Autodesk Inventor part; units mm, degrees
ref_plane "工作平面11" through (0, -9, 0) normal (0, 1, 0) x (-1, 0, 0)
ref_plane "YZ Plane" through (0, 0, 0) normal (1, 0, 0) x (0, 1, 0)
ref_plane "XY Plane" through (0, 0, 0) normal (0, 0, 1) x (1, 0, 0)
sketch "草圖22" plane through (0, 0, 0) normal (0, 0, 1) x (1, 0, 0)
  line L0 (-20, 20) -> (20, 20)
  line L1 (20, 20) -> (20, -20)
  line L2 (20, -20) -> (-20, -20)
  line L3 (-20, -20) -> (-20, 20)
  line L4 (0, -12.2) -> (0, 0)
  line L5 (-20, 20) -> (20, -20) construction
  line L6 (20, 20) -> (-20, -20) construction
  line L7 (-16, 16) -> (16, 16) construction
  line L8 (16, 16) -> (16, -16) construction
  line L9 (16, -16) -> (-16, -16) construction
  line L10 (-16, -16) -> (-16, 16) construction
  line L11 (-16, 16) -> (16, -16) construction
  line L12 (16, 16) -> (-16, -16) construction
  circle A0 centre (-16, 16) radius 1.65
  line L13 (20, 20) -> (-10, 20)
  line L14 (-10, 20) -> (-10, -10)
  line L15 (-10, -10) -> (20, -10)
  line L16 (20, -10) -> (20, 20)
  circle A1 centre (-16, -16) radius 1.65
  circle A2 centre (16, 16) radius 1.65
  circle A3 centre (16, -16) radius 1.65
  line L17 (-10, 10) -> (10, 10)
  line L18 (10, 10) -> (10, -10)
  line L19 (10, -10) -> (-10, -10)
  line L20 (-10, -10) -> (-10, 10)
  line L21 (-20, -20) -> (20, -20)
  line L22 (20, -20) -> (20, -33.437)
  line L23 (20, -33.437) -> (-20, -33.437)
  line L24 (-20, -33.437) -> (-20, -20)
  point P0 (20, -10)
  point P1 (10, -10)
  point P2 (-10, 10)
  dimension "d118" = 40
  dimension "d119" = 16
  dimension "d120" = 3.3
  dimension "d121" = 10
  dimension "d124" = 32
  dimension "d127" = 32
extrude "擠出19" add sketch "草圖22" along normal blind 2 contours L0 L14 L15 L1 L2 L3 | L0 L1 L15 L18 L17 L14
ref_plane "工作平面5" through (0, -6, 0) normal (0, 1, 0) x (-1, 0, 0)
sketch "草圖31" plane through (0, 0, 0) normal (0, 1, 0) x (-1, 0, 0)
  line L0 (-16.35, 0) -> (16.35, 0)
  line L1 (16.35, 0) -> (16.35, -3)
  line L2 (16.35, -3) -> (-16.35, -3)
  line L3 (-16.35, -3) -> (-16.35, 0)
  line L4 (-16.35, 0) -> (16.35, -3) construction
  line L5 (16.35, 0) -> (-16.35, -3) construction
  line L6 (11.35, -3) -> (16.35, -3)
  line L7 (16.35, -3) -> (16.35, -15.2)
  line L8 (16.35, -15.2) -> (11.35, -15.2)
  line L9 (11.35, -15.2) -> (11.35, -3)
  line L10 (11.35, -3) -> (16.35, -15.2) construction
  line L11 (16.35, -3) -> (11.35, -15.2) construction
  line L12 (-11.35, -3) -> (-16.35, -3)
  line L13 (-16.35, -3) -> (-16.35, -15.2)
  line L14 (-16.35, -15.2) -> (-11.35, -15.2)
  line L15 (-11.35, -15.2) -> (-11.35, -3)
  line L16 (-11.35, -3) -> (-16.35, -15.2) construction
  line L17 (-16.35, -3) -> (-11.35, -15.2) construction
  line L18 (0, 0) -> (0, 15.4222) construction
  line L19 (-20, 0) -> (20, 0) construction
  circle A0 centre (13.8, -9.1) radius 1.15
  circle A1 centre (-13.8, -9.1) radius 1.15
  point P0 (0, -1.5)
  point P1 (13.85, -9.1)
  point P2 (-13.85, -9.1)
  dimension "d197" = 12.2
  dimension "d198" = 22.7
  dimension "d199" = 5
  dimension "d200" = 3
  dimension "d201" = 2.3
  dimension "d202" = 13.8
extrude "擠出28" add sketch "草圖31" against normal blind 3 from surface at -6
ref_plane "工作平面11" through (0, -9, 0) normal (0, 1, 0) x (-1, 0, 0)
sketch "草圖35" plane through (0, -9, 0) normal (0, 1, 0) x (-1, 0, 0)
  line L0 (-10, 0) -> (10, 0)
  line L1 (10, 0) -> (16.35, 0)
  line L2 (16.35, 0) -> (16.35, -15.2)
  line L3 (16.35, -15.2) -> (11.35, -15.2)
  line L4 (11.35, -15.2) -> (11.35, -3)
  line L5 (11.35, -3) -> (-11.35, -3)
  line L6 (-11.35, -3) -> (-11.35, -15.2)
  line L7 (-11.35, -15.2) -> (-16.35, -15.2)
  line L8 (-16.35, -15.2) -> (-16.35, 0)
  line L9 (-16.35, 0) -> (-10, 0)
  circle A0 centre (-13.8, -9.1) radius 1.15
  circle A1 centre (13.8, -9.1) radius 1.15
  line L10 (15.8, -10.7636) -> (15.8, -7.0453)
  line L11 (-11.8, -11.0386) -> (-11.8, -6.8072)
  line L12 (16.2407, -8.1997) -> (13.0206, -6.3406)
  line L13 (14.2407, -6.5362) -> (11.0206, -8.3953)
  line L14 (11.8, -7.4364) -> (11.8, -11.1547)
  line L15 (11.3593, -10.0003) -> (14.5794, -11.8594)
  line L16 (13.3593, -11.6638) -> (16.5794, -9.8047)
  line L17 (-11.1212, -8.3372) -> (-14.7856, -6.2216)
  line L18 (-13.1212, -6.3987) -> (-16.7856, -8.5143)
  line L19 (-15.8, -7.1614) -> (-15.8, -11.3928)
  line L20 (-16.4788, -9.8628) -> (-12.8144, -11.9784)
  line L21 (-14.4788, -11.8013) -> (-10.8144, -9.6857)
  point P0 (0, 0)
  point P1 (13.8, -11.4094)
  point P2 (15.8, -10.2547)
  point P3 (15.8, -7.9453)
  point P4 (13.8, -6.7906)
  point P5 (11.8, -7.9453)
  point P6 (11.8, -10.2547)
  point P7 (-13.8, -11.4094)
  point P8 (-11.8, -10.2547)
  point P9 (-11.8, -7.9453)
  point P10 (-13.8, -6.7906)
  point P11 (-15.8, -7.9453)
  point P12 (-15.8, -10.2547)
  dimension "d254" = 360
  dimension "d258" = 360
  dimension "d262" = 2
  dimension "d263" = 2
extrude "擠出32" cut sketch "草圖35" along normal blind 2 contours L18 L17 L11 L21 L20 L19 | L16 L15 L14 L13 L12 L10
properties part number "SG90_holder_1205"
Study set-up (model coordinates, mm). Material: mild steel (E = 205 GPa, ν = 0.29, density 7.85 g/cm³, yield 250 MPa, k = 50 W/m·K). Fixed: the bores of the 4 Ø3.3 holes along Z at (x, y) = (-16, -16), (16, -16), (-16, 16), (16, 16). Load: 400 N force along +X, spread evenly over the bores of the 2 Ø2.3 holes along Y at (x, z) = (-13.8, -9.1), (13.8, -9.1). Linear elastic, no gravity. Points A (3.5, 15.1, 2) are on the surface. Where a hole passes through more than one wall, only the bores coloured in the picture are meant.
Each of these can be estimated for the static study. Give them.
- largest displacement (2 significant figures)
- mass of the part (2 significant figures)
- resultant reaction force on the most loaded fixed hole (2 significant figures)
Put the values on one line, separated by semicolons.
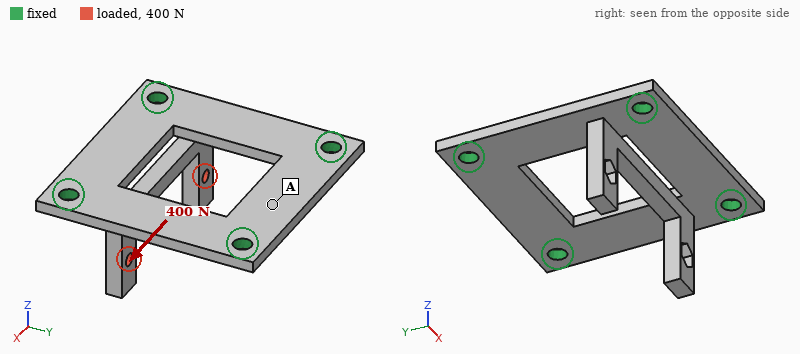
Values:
47 µm; 23 g; 190 N
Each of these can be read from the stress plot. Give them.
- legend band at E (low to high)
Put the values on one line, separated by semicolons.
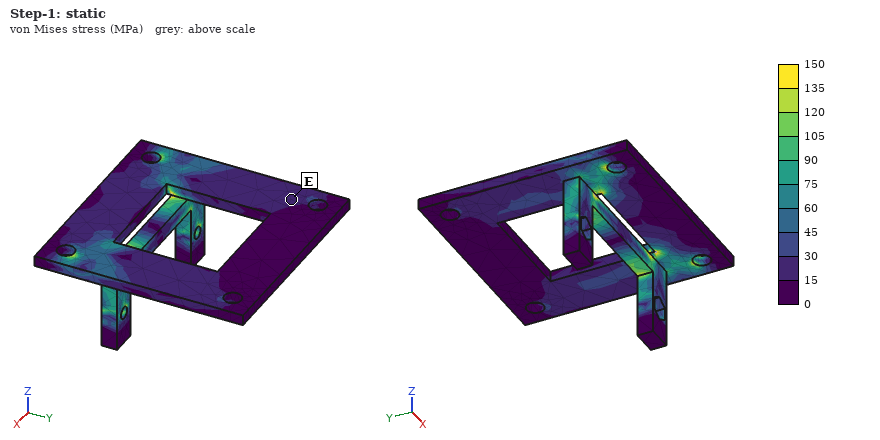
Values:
15 to 30 MPa
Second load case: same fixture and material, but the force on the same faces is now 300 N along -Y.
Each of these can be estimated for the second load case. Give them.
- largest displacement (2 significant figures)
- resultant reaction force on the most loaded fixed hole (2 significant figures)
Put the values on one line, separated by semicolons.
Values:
78 µm; 120 N
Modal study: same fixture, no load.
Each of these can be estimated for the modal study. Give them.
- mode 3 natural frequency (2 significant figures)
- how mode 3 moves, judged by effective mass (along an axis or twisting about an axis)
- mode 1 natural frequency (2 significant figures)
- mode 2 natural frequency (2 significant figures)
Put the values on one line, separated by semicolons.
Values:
9600 Hz; along Z; 6500 Hz; 7200 Hz
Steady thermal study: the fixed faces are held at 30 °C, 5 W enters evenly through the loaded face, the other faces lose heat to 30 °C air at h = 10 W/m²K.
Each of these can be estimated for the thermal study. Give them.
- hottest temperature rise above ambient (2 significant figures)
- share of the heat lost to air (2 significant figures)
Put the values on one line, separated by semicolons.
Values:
58 K; 7.6 %
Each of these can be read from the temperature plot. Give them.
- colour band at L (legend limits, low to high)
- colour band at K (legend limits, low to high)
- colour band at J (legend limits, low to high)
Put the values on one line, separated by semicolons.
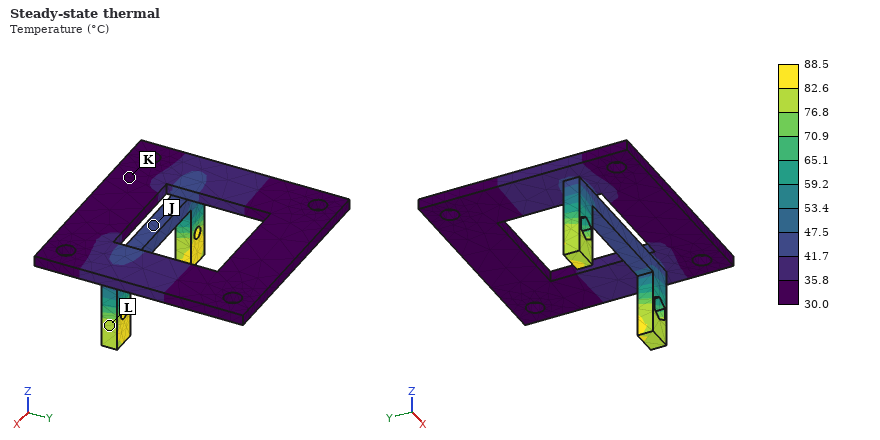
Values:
76.8 to 82.6 °C; 30.0 to 35.8 °C; 41.7 to 47.5 °C
